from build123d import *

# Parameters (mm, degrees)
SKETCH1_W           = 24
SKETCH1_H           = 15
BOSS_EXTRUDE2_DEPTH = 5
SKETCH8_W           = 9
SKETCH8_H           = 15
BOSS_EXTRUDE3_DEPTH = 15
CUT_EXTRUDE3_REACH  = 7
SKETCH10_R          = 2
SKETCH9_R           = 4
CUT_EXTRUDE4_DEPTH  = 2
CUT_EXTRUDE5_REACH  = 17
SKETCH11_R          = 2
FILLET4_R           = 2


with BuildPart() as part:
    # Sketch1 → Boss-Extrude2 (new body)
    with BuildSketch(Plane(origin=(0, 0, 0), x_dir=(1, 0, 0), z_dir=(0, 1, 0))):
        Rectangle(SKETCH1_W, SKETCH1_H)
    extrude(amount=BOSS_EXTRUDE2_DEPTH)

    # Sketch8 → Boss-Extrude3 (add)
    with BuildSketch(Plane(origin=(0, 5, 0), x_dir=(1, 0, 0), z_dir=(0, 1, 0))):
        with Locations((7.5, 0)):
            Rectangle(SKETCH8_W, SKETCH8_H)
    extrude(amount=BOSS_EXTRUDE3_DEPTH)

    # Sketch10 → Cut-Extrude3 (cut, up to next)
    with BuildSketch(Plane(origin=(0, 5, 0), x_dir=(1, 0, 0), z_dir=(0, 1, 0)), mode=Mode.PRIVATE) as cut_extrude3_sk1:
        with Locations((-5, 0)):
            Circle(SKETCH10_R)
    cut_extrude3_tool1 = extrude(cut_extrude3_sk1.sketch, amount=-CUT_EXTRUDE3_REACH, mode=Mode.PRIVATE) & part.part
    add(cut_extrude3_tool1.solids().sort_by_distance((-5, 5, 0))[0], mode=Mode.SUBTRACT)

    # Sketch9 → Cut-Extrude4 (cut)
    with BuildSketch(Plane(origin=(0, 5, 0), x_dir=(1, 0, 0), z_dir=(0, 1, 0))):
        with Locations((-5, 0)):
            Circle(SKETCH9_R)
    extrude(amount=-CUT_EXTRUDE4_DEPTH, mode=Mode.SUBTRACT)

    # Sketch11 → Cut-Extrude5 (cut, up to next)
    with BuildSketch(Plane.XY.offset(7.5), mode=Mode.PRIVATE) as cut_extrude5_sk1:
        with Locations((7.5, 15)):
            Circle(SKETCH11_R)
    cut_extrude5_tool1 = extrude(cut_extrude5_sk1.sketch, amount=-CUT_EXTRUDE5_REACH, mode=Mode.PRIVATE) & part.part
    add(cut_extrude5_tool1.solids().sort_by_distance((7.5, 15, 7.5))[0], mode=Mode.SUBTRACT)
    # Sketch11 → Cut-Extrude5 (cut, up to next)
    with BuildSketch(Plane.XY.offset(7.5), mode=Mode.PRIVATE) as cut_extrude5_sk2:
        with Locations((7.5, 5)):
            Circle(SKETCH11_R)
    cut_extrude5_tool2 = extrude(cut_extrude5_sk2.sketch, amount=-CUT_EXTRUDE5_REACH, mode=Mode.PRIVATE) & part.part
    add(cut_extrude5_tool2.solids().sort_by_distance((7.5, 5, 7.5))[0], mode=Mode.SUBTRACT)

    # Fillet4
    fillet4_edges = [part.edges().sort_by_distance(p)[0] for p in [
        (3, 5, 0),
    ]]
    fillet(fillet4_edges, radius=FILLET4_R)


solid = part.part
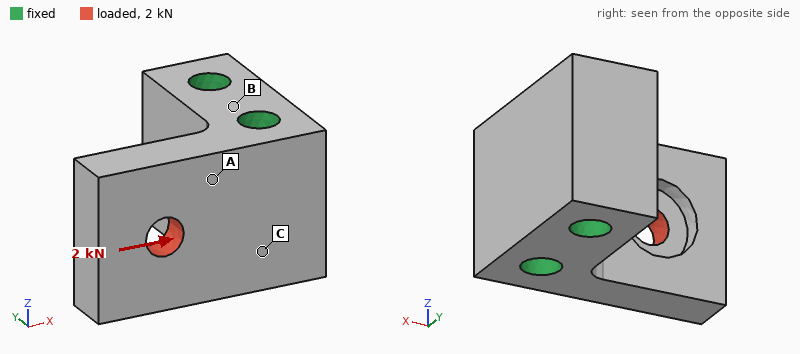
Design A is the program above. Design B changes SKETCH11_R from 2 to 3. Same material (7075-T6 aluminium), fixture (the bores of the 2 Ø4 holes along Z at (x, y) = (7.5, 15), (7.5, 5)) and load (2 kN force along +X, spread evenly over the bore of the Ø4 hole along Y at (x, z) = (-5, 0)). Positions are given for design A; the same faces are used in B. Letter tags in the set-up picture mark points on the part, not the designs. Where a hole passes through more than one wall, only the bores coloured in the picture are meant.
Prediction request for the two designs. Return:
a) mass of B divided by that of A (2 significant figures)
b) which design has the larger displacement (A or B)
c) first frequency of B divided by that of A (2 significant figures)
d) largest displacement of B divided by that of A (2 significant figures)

0.86
A
1.1
0.86
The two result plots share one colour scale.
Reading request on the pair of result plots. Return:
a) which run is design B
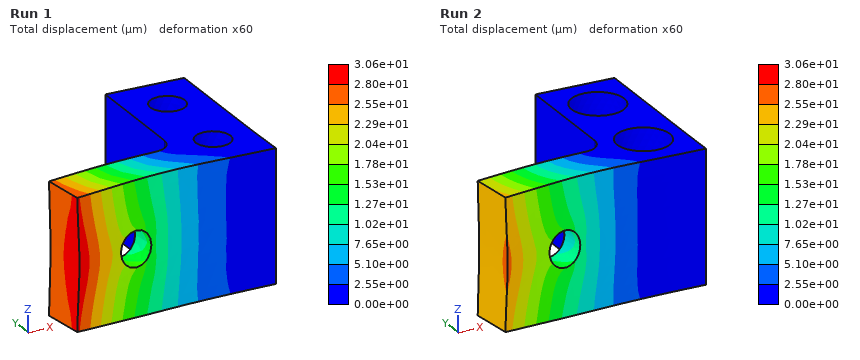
Run 2
